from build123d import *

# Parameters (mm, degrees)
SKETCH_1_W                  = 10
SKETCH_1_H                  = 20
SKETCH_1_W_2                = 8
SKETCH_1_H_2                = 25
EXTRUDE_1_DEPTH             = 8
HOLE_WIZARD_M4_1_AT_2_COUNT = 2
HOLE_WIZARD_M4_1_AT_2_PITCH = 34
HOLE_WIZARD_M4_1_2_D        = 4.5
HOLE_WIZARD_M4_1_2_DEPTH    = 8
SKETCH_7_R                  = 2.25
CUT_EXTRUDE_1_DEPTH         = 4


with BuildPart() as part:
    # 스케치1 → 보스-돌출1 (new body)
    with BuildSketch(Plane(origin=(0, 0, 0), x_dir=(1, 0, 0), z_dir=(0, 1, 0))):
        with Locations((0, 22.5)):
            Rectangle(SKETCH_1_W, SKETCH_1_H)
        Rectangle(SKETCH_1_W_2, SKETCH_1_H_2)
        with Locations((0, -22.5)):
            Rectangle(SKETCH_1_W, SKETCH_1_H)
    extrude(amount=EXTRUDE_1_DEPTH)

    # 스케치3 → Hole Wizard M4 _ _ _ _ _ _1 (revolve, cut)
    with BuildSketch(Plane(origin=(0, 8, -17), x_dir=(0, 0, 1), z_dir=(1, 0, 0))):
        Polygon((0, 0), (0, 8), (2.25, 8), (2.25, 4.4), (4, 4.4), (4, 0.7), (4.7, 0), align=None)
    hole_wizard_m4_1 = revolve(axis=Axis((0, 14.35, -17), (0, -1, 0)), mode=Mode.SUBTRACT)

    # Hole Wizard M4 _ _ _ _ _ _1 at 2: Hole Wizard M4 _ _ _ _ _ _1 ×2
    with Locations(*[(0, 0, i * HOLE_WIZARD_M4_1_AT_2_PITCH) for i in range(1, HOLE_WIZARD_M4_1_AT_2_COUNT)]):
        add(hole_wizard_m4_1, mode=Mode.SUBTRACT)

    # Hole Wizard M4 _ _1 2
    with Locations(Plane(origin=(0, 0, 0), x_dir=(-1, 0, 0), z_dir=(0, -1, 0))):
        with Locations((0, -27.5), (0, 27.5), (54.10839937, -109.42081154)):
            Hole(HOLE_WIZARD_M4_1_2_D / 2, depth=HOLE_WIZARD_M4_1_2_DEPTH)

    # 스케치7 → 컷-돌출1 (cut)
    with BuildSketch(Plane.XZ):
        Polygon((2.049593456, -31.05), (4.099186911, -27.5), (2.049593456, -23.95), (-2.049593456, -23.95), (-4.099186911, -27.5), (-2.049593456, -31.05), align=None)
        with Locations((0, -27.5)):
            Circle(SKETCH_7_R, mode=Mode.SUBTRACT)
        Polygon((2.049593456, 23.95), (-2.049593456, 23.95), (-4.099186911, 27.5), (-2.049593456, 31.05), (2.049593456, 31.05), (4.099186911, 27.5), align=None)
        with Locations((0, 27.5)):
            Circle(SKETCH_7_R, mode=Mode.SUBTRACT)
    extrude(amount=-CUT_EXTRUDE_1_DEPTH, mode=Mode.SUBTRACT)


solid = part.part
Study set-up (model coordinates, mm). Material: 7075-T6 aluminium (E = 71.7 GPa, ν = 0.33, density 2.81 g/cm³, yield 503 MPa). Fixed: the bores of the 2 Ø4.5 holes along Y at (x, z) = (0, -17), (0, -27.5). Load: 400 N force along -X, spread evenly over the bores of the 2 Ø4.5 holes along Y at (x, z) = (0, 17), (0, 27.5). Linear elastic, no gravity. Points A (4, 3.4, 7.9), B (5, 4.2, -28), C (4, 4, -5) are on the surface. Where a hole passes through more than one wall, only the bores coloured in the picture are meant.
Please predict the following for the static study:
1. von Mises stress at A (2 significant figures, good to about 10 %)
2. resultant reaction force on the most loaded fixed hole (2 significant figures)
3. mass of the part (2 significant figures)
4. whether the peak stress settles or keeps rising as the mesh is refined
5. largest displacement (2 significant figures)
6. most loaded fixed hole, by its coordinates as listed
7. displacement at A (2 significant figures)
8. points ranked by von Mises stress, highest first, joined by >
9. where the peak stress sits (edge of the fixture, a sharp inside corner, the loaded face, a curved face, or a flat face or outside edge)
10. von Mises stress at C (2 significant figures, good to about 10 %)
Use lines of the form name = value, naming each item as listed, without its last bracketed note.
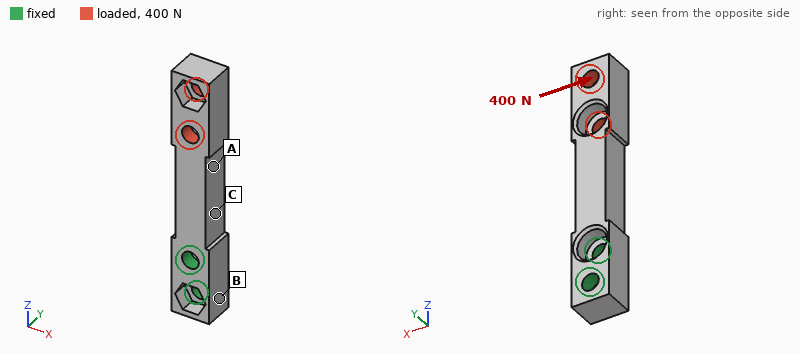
von Mises stress at A = 72 MPa
resultant reaction force on the most loaded fixed hole = 830 N
mass of the part = 11 g
whether the peak stress settles or keeps rising as the mesh is refined = keeps rising
largest displacement = 0.54 mm
most loaded fixed hole, by its coordinates as listed = (0, -17)
displacement at A = 0.19 mm
points ranked by von Mises stress, highest first, joined by > = C > A > B
where the peak stress sits = edge of the fixture
von Mises stress at C = 130 MPa
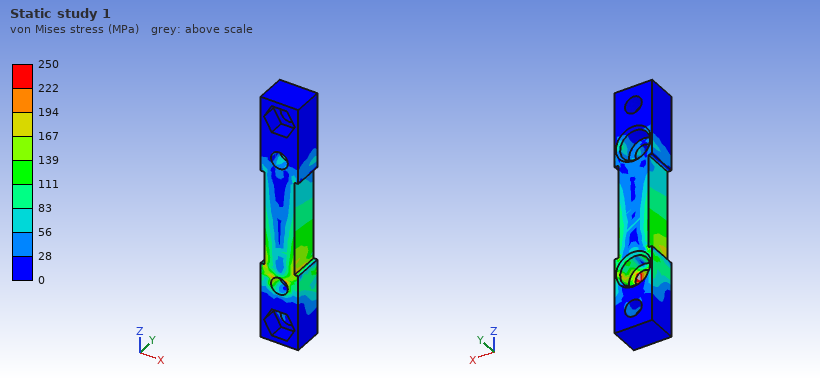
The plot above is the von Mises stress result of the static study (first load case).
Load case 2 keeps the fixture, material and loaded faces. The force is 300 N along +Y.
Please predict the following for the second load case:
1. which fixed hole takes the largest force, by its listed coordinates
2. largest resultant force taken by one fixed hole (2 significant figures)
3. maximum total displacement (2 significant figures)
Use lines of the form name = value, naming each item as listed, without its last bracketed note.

which fixed hole takes the largest force, by its listed coordinates = (0, -17)
largest resultant force taken by one fixed hole = 820 N
maximum total displacement = 0.56 mm
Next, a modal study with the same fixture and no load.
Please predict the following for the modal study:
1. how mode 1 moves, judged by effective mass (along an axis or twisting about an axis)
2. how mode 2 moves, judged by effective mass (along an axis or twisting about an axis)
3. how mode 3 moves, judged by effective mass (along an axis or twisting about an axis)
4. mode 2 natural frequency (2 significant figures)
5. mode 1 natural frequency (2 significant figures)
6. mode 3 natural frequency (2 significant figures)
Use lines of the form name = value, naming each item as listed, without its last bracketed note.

how mode 1 moves, judged by effective mass = along Y
how mode 2 moves, judged by effective mass = along X
how mode 3 moves, judged by effective mass = twisting about Z
mode 2 natural frequency = 2600 Hz
mode 1 natural frequency = 2200 Hz
mode 3 natural frequency = 12 kHz
